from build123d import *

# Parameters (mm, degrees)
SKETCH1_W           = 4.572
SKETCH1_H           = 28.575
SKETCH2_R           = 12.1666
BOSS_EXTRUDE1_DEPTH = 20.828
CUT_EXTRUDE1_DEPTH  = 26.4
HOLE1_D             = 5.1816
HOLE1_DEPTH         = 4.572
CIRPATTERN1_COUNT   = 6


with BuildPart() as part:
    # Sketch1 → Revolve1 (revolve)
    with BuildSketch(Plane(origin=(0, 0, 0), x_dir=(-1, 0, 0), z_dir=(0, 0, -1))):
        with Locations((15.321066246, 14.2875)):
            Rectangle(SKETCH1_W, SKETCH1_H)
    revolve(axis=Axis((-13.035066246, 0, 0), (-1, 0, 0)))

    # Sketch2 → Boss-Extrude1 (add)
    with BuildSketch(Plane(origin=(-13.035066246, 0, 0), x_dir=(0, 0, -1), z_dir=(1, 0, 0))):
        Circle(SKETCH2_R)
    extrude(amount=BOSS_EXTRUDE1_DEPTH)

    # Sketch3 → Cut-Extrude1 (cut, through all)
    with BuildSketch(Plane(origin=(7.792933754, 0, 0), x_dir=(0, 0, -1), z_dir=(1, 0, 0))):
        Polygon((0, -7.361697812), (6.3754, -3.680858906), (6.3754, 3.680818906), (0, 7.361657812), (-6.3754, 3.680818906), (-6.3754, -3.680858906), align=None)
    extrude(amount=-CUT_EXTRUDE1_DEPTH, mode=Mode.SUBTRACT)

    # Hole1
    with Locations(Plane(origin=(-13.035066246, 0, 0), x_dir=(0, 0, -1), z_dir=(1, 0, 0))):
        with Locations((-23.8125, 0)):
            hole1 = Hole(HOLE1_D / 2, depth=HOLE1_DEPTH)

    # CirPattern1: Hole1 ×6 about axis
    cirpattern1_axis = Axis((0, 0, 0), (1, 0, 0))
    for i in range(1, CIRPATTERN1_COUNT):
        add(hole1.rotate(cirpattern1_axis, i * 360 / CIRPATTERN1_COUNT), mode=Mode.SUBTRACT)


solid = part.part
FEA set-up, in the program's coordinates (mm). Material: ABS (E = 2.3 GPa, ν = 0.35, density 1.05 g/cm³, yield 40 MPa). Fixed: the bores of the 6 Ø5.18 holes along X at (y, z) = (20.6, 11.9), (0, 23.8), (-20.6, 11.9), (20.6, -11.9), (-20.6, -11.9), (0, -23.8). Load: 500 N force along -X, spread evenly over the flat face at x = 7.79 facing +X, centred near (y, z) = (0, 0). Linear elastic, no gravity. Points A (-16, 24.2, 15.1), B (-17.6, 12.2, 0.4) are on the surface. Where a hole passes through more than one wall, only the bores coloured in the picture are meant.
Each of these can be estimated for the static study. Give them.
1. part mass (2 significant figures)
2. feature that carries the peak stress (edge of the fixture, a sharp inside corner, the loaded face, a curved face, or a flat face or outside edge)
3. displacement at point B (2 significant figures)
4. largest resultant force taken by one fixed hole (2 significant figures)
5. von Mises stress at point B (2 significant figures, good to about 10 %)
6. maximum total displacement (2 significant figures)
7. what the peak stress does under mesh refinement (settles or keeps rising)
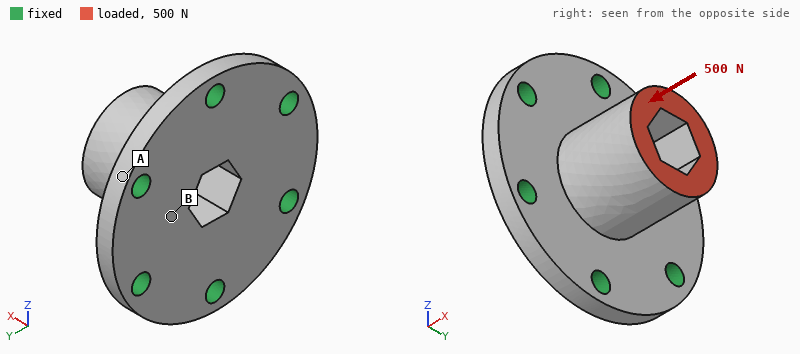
18 g
edge of the fixture
67 µm
93 N
4.3 MPa
88 µm
keeps rising
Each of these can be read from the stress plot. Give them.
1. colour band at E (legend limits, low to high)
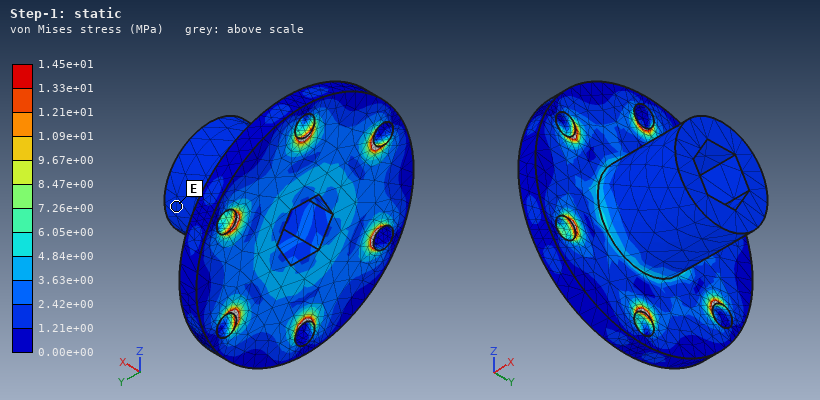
1.21e+00 to 2.42e+00 MPa
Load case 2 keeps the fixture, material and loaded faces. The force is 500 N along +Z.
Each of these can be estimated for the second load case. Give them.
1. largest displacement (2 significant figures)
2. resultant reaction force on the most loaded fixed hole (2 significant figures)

0.40 mm
250 N
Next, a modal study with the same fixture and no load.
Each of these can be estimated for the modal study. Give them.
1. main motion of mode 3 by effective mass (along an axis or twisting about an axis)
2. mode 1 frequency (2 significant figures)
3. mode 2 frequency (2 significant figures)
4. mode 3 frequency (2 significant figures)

along X
3400 Hz
3400 Hz
4100 Hz
